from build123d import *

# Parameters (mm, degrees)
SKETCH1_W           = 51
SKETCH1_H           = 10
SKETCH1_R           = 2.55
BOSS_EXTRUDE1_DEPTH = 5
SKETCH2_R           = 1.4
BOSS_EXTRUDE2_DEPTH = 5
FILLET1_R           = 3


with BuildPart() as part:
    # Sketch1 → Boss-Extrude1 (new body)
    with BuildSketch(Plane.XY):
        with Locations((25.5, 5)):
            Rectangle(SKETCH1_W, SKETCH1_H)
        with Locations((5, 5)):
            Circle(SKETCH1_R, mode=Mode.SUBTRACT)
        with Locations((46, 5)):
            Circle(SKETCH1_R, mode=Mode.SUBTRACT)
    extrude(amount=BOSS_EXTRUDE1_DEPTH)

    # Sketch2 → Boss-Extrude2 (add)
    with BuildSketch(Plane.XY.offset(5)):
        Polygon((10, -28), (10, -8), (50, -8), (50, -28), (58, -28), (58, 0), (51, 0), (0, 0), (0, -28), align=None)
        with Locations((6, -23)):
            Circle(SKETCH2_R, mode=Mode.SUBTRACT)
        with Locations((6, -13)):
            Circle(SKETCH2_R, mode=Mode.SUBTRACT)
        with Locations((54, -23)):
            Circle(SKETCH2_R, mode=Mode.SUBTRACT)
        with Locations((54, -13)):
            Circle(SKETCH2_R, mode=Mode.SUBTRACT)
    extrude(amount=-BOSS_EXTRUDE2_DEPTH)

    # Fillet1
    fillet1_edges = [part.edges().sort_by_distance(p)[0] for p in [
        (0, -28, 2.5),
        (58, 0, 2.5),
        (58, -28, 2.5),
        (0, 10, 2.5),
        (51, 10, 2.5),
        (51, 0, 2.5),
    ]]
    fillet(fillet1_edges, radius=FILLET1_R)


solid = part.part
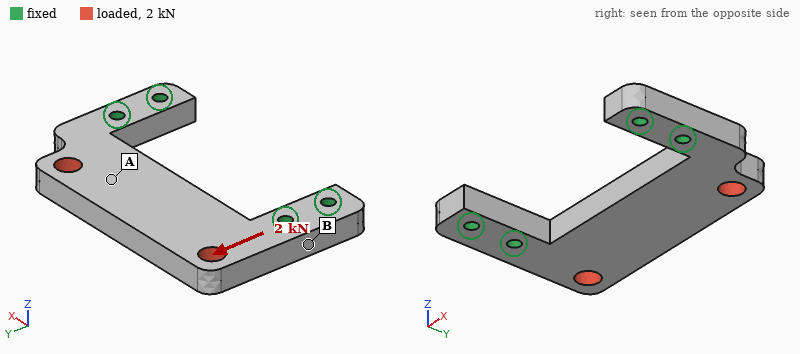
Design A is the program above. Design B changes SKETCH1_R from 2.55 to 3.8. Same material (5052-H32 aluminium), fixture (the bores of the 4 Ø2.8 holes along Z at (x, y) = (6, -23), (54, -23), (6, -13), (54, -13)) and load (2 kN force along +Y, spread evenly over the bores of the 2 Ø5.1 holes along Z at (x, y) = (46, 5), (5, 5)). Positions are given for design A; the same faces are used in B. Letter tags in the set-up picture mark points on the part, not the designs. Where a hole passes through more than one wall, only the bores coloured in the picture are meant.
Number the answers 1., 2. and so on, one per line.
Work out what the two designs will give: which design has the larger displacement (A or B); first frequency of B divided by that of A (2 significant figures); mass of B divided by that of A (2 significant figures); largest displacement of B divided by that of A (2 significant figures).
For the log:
1. B
2. 1.0
3. 0.96
4. 1.5
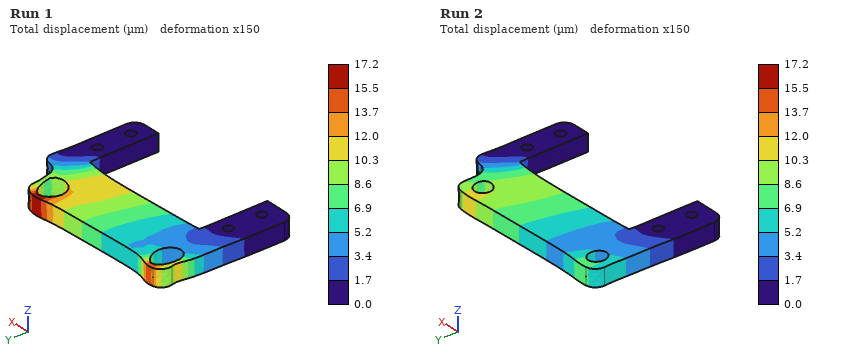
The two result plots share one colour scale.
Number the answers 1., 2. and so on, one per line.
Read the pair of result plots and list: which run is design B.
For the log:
1. Run 1
